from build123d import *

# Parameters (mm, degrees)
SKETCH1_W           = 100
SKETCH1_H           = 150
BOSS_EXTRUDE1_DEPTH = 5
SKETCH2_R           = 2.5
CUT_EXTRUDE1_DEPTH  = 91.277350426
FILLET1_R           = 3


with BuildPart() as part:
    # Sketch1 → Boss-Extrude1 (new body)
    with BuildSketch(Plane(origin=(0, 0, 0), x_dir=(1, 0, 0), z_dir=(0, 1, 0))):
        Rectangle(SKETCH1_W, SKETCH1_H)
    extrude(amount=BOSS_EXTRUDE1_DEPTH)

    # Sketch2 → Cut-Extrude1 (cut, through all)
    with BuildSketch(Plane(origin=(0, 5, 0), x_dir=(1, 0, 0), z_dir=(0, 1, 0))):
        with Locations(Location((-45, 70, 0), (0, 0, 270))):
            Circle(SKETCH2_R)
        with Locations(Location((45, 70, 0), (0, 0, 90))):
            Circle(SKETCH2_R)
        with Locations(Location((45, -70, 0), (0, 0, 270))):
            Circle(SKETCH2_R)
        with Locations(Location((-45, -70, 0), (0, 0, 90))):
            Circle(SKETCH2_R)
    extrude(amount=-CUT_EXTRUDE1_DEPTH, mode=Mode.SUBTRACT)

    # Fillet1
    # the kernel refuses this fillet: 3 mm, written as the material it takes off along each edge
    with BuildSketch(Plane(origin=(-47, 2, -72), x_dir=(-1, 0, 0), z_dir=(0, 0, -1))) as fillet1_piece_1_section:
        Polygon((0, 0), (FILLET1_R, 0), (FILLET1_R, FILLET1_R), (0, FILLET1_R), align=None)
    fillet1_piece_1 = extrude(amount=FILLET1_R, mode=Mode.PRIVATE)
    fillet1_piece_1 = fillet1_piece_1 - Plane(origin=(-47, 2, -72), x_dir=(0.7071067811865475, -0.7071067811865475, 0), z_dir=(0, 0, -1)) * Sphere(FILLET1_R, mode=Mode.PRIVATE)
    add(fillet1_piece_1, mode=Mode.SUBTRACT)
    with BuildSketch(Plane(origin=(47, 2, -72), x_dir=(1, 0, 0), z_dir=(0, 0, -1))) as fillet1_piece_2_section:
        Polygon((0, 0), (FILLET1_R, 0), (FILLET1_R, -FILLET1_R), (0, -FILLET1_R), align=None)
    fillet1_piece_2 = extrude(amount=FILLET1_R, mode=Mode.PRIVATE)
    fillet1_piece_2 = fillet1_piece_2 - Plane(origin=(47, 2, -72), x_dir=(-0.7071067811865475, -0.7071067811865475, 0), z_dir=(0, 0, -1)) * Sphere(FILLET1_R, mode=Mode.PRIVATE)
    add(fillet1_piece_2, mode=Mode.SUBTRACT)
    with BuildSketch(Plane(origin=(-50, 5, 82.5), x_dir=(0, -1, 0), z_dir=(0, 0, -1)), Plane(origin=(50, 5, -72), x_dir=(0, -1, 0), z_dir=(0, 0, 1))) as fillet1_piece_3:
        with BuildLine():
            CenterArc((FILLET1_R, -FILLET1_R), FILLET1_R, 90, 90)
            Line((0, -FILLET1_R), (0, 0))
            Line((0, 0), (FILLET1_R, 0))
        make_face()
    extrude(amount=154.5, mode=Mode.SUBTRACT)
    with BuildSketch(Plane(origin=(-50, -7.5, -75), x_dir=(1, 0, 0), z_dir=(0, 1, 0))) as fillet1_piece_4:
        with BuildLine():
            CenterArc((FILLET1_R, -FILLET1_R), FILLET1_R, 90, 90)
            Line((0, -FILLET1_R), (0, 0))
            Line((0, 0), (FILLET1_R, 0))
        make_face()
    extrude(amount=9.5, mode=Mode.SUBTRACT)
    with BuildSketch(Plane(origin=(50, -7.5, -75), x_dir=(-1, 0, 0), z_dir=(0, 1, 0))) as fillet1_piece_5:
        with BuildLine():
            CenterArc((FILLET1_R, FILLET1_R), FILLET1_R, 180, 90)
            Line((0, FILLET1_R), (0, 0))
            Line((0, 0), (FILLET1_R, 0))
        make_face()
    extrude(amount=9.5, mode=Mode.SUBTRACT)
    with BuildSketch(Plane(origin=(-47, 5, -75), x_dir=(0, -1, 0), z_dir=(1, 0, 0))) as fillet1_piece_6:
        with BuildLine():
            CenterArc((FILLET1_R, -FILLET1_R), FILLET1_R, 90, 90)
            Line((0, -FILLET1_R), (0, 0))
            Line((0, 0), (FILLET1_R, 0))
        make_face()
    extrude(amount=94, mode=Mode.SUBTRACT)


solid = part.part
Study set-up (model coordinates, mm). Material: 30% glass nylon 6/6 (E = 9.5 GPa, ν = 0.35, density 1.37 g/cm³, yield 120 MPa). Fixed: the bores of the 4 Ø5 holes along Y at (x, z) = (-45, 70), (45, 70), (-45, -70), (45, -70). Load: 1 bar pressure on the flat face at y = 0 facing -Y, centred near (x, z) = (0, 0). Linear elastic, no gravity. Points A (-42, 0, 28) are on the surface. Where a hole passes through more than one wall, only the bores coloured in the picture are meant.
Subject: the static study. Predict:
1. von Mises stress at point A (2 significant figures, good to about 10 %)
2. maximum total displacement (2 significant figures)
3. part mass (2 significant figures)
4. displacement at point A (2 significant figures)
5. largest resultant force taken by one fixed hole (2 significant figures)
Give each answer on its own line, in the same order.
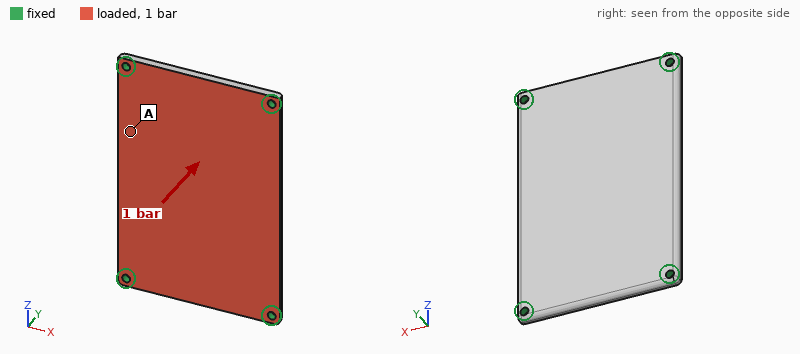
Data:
19 MPa
1.8 mm
100 g
1.2 mm
370 N
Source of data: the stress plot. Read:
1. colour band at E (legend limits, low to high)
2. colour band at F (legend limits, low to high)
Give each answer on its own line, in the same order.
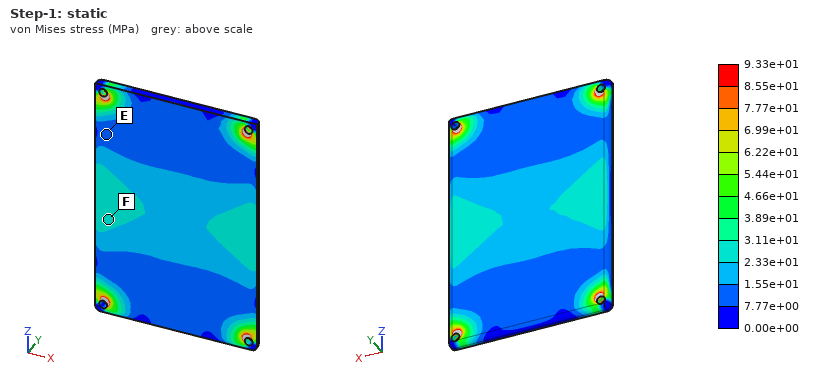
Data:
7.77e+00 to 1.55e+01 MPa
2.33e+01 to 3.11e+01 MPa
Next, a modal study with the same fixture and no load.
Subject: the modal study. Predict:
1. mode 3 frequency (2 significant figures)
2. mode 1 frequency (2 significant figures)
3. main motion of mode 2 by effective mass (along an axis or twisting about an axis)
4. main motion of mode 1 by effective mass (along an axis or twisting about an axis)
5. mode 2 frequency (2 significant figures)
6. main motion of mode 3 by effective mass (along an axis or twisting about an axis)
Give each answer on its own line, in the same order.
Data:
1300 Hz
530 Hz
twisting about Z
along Y
910 Hz
twisting about X
